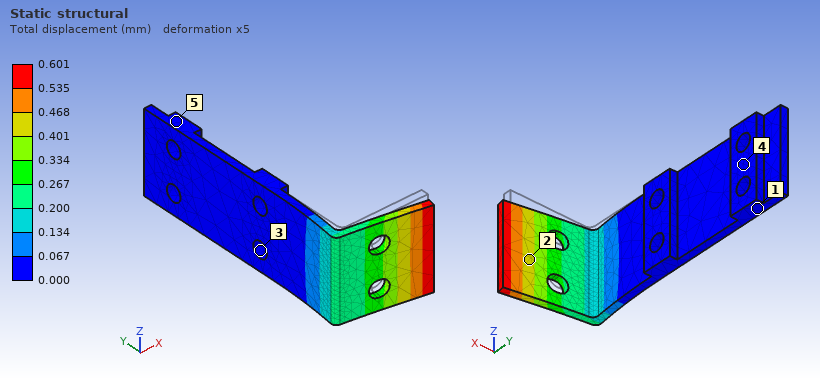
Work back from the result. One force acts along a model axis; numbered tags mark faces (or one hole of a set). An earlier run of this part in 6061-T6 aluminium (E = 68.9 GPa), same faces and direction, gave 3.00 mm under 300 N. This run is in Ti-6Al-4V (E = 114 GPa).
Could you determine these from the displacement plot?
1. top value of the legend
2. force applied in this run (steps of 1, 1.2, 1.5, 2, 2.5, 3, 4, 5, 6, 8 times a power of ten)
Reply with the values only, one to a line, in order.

0.601 mm
100 N
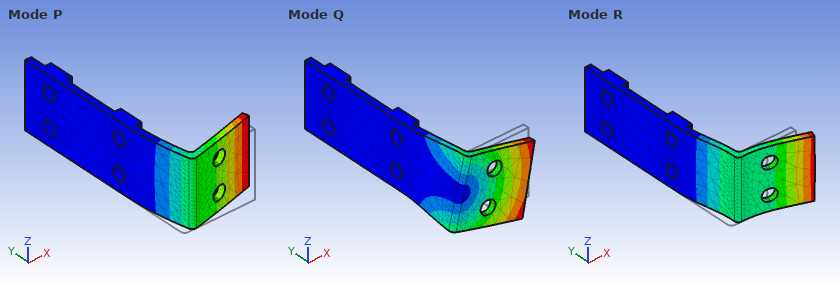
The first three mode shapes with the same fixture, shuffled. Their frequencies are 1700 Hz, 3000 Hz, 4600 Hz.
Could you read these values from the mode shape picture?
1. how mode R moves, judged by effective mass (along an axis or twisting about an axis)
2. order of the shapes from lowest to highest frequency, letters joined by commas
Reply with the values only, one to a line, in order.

along X
P, Q, R
